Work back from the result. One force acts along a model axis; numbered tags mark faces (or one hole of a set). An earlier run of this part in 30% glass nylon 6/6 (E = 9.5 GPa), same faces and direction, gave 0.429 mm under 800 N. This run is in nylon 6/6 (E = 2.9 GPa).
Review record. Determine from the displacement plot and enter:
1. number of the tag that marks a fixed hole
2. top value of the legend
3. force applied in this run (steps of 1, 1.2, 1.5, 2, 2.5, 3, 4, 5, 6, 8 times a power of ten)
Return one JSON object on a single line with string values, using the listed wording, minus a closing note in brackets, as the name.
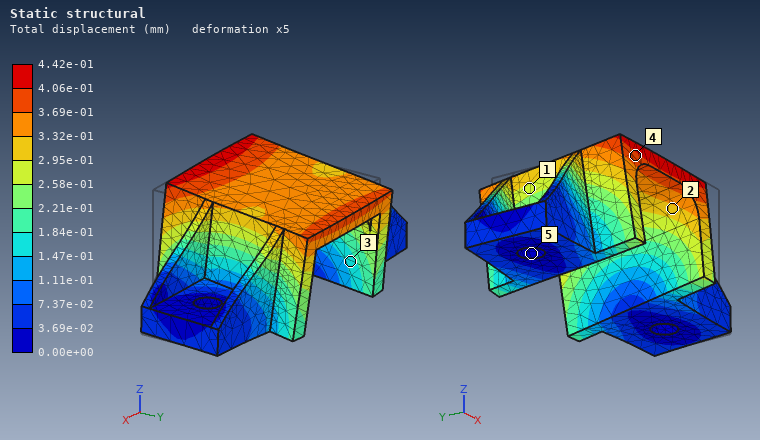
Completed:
{"number of the tag that marks a fixed hole": "5", "top value of the legend": "4.42e-01 mm", "force applied in this run": "250 N"}
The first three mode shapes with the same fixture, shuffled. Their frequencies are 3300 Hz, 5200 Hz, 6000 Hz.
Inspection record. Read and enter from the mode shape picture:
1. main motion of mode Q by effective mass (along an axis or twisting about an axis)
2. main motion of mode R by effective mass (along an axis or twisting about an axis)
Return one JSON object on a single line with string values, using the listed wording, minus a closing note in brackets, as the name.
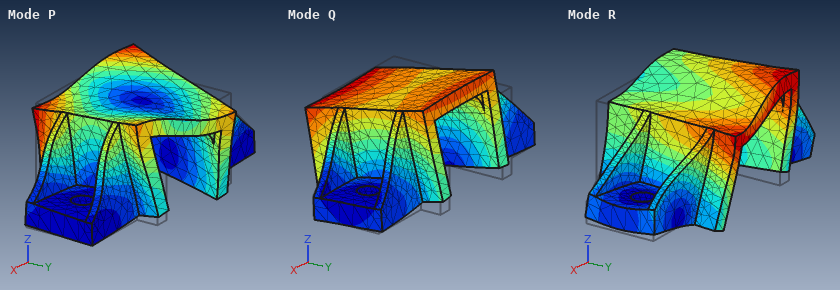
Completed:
{"main motion of mode Q by effective mass": "along Y", "main motion of mode R by effective mass": "along X"}
